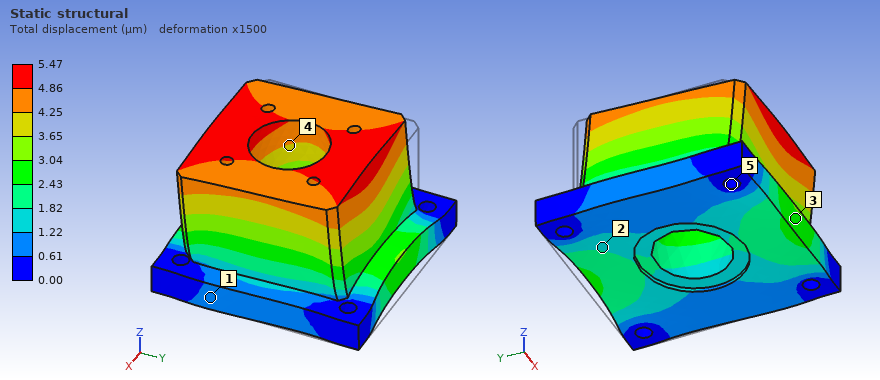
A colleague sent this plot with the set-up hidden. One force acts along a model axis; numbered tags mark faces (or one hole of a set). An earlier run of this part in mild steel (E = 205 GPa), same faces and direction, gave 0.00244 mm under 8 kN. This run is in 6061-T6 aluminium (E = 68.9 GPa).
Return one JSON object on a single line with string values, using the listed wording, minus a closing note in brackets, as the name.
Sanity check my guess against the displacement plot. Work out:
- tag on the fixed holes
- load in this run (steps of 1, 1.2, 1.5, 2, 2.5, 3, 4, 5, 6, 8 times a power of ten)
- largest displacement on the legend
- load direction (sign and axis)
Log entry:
{"tag on the fixed holes": "5", "load in this run": "6 kN", "largest displacement on the legend": "5.47 µm", "load direction": "-Y"}
